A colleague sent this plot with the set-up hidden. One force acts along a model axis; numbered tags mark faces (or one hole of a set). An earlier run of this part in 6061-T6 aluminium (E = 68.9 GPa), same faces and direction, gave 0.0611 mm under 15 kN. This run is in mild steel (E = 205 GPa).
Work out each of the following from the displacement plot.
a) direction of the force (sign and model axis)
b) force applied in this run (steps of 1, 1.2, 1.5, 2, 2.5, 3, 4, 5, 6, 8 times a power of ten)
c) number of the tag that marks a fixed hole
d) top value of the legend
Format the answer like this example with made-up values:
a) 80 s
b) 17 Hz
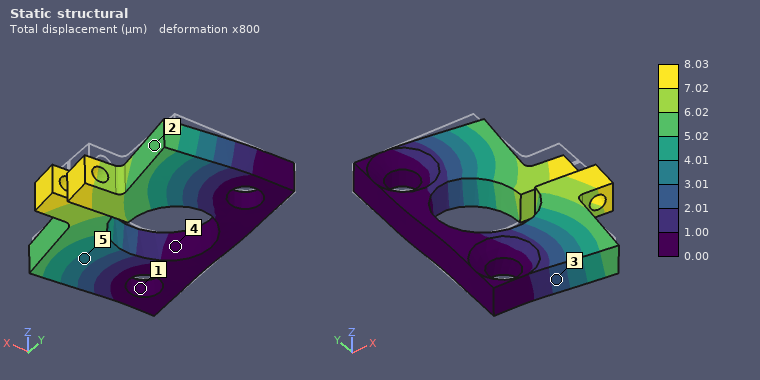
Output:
a) -Y
b) 6 kN
c) 1
d) 8.03 µm
